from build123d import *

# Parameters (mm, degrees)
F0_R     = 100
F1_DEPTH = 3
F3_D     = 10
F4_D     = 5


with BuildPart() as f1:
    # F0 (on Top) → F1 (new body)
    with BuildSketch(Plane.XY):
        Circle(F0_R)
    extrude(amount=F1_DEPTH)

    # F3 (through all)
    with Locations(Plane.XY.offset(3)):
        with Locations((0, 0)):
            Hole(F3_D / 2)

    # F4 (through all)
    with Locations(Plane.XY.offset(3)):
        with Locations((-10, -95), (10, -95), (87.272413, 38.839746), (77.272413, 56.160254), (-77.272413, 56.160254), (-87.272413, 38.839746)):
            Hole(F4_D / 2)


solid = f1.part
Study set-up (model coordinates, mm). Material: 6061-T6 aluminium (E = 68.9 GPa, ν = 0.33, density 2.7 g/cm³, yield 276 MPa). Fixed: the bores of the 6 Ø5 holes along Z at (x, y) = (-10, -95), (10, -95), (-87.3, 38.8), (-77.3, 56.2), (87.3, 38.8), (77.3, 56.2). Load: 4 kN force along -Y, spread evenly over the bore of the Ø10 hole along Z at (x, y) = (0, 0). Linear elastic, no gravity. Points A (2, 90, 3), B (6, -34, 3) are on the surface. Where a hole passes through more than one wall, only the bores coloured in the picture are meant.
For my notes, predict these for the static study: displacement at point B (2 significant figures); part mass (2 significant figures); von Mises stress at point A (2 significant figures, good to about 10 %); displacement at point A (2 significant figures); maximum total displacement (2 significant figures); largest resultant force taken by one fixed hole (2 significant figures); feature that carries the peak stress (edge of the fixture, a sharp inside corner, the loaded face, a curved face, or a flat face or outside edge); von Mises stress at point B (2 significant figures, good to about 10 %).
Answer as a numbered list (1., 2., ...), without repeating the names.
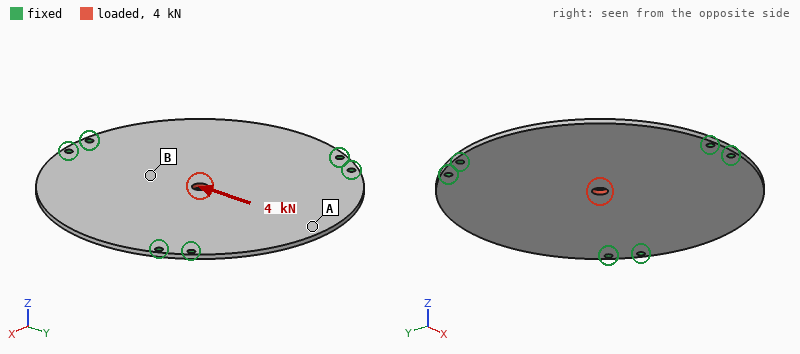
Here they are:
1. 12 µm
2. 250 g
3. 5.4 MPa
4. 12 µm
5. 23 µm
6. 830 N
7. the loaded face
8. 15 MPa
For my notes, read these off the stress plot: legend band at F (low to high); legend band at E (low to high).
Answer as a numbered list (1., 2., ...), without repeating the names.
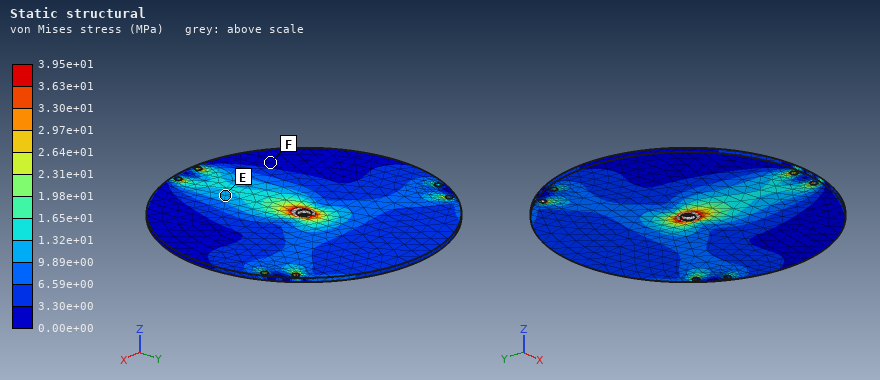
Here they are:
1. 0.00e+00 to 3.30e+00 MPa
2. 9.89e+00 to 1.32e+01 MPa
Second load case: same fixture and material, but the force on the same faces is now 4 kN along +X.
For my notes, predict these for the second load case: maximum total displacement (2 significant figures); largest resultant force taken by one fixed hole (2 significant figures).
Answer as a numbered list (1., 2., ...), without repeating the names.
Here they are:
1. 23 µm
2. 830 N
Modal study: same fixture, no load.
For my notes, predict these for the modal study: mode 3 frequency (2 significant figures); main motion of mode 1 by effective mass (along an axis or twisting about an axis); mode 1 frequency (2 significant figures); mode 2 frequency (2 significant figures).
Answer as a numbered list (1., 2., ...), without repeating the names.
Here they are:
1. 530 Hz
2. along Z
3. 500 Hz
4. 530 Hz
